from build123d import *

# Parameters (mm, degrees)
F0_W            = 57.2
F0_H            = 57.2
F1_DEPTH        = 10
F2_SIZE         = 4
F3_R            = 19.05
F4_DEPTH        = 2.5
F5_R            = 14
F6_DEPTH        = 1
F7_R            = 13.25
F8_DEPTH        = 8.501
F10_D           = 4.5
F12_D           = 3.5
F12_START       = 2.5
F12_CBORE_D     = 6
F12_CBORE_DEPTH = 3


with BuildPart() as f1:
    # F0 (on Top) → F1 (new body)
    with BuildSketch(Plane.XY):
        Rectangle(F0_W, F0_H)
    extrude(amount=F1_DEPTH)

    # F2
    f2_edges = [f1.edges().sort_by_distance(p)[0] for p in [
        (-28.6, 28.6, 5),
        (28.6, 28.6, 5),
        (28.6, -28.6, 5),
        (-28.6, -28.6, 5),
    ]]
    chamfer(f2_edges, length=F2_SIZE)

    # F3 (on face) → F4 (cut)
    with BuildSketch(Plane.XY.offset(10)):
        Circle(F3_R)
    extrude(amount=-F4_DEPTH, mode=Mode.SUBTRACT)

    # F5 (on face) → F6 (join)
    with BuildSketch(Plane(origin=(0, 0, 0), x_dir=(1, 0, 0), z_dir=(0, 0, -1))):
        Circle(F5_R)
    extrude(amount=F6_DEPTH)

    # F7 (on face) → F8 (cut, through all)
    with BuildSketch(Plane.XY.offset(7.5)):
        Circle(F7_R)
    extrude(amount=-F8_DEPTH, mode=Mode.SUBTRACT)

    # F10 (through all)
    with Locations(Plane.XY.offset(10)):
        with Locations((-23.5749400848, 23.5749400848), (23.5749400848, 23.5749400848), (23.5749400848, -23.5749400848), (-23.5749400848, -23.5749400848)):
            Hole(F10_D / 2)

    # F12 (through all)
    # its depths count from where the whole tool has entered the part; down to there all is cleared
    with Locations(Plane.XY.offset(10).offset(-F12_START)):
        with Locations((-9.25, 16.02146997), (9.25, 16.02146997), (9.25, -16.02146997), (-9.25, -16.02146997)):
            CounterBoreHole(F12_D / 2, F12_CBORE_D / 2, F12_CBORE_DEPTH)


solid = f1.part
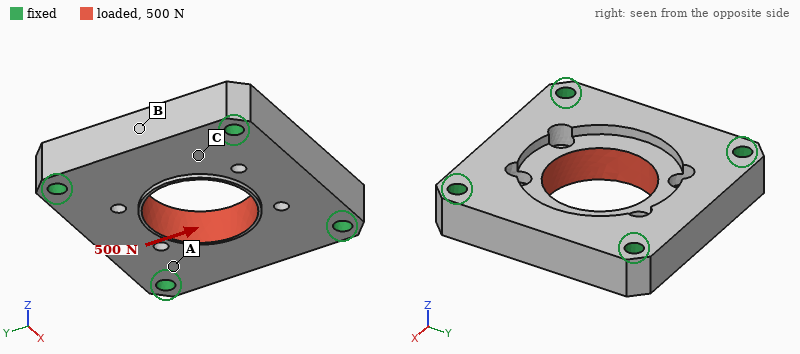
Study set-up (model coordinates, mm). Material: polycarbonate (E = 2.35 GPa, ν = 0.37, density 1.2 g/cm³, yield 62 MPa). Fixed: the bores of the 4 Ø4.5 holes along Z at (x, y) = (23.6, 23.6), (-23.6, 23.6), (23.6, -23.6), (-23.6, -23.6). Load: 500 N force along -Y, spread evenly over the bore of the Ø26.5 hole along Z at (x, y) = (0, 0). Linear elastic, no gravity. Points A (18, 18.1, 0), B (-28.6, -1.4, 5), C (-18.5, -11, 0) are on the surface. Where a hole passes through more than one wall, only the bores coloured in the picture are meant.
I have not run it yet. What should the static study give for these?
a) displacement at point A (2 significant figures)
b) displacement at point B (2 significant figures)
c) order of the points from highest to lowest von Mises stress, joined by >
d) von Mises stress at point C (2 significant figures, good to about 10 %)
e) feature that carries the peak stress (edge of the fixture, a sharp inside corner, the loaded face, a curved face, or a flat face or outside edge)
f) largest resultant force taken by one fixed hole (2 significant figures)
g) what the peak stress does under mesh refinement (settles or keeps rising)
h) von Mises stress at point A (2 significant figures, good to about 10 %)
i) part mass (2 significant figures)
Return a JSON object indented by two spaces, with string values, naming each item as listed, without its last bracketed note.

{
  "displacement at point A": "5.3 µm",
  "displacement at point B": "4.9 µm",
  "order of the points from highest to lowest von Mises stress, joined by >": "A > C > B",
  "von Mises stress at point C": "0.81 MPa",
  "feature that carries the peak stress": "edge of the fixture",
  "largest resultant force taken by one fixed hole": "140 N",
  "what the peak stress does under mesh refinement": "keeps rising",
  "von Mises stress at point A": "1.3 MPa",
  "part mass": "29 g"
}
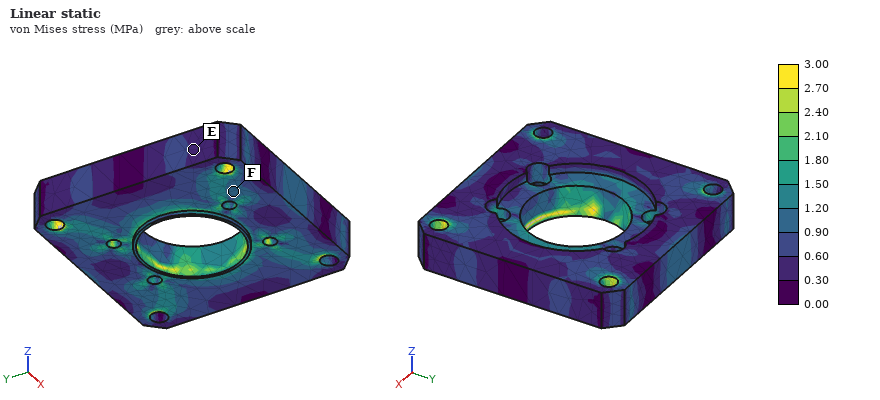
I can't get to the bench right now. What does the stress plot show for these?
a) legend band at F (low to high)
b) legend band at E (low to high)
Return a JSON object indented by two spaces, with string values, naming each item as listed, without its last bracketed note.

{
  "legend band at F": "0.90 to 1.20 MPa",
  "legend band at E": "0.30 to 0.60 MPa"
}
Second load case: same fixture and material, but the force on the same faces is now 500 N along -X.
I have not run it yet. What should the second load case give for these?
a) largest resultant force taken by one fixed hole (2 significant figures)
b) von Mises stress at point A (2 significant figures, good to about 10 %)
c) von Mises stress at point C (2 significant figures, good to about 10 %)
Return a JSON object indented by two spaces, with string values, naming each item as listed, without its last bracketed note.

{
  "largest resultant force taken by one fixed hole": "140 N",
  "von Mises stress at point A": "1.3 MPa",
  "von Mises stress at point C": "1.2 MPa"
}
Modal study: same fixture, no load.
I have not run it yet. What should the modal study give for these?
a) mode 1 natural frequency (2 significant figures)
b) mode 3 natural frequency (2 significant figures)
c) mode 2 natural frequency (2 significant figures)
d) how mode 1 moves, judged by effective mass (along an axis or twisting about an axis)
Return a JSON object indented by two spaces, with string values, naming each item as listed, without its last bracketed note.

{
  "mode 1 natural frequency": "4200 Hz",
  "mode 3 natural frequency": "5200 Hz",
  "mode 2 natural frequency": "5200 Hz",
  "how mode 1 moves, judged by effective mass": "along Z"
}
